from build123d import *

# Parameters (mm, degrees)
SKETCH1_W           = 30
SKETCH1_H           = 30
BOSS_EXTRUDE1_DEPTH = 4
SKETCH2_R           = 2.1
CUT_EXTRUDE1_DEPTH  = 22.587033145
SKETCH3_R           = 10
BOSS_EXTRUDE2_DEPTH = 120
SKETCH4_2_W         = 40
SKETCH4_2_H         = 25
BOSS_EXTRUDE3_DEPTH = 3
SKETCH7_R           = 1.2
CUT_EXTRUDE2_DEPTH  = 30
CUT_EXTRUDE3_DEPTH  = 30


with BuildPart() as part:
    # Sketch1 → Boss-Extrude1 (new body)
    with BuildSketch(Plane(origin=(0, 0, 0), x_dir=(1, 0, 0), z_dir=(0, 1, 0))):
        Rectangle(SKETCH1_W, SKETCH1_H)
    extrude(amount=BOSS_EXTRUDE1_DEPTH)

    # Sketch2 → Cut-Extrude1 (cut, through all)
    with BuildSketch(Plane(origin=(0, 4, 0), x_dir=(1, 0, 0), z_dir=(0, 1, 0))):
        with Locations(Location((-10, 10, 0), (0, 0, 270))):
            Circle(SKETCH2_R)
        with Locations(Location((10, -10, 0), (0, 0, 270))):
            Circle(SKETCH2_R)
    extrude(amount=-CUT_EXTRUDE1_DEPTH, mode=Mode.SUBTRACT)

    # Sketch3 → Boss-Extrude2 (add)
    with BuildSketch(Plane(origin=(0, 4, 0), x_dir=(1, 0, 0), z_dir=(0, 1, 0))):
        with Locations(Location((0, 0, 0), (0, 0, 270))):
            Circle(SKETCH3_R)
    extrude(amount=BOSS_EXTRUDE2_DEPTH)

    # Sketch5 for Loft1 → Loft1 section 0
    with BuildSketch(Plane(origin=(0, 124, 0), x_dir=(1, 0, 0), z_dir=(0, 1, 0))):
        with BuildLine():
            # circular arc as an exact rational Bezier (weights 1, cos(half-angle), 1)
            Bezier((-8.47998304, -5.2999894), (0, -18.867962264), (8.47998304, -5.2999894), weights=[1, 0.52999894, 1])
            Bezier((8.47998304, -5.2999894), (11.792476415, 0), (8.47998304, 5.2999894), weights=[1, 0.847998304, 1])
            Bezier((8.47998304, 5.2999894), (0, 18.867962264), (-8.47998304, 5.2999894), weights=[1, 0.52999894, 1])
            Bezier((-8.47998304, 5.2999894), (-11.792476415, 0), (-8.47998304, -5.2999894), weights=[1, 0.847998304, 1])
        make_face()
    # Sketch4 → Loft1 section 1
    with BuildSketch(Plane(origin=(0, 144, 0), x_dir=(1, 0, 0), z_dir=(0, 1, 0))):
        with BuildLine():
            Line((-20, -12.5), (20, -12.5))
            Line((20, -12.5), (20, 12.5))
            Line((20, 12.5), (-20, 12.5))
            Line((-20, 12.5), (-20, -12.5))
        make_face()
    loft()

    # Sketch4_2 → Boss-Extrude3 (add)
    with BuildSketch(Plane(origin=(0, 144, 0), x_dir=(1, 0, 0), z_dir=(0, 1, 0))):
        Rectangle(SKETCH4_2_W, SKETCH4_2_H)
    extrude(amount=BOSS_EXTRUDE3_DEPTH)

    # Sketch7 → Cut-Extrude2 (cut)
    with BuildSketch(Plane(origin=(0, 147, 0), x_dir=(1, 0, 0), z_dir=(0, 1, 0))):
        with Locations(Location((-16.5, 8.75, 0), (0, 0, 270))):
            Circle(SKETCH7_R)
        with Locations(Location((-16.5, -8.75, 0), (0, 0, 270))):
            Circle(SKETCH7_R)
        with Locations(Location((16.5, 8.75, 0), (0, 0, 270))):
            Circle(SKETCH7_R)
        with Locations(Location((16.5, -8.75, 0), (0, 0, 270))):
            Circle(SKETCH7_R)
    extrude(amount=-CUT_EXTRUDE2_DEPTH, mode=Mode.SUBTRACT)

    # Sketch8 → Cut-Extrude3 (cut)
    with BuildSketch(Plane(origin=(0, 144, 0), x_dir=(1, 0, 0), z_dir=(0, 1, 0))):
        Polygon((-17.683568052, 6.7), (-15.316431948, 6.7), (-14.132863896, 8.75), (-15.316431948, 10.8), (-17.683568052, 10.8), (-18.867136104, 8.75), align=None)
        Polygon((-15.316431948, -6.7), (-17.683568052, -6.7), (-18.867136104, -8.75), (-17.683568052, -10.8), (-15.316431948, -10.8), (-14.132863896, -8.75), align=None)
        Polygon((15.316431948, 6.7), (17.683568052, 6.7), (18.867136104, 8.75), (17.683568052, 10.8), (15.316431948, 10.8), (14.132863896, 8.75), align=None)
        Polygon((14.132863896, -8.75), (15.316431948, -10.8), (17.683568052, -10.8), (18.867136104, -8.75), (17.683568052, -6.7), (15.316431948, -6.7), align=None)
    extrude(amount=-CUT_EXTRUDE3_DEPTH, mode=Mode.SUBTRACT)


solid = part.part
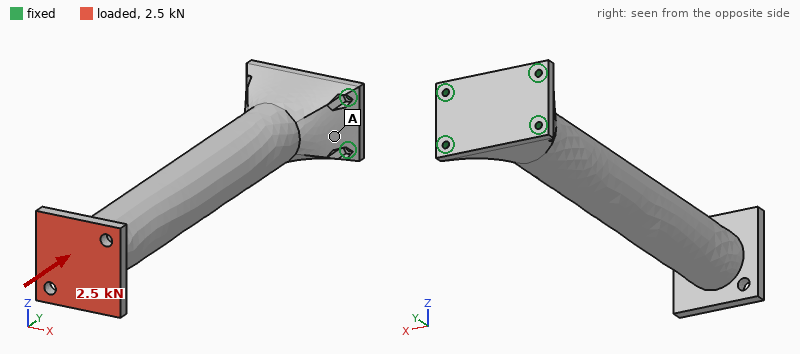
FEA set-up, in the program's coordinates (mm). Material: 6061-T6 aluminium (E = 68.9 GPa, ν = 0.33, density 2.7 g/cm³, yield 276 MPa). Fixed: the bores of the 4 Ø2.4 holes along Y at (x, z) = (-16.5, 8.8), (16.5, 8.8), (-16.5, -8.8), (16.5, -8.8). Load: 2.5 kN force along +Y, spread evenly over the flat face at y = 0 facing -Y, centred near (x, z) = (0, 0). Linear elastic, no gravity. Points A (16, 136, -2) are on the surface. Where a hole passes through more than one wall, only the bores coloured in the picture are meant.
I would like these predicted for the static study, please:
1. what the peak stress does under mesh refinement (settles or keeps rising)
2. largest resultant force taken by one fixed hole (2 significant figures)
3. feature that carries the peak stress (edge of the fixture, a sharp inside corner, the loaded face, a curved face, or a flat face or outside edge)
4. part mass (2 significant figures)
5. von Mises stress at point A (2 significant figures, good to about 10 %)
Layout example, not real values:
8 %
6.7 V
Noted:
keeps rising
700 N
edge of the fixture
150 g
8.2 MPa
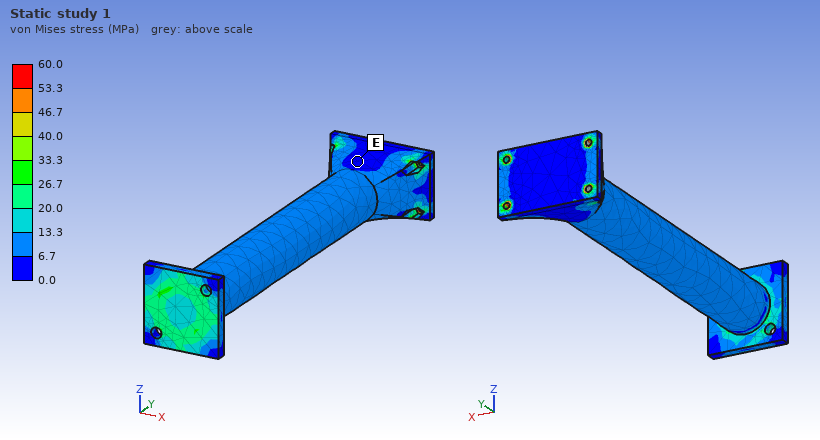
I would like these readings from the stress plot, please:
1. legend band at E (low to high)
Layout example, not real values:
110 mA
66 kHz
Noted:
0.0 to 6.7 MPa
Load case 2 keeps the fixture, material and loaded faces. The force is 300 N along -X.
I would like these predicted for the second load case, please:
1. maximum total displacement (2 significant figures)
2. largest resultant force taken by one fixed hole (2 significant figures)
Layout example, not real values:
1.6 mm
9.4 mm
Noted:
0.46 mm
700 N
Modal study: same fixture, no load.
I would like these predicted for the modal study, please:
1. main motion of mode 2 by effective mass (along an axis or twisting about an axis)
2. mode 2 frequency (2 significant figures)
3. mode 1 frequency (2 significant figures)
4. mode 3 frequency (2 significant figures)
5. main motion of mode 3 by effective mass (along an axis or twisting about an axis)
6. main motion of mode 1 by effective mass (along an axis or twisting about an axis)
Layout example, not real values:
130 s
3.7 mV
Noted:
along X
700 Hz
600 Hz
3500 Hz
along Z
along Z
